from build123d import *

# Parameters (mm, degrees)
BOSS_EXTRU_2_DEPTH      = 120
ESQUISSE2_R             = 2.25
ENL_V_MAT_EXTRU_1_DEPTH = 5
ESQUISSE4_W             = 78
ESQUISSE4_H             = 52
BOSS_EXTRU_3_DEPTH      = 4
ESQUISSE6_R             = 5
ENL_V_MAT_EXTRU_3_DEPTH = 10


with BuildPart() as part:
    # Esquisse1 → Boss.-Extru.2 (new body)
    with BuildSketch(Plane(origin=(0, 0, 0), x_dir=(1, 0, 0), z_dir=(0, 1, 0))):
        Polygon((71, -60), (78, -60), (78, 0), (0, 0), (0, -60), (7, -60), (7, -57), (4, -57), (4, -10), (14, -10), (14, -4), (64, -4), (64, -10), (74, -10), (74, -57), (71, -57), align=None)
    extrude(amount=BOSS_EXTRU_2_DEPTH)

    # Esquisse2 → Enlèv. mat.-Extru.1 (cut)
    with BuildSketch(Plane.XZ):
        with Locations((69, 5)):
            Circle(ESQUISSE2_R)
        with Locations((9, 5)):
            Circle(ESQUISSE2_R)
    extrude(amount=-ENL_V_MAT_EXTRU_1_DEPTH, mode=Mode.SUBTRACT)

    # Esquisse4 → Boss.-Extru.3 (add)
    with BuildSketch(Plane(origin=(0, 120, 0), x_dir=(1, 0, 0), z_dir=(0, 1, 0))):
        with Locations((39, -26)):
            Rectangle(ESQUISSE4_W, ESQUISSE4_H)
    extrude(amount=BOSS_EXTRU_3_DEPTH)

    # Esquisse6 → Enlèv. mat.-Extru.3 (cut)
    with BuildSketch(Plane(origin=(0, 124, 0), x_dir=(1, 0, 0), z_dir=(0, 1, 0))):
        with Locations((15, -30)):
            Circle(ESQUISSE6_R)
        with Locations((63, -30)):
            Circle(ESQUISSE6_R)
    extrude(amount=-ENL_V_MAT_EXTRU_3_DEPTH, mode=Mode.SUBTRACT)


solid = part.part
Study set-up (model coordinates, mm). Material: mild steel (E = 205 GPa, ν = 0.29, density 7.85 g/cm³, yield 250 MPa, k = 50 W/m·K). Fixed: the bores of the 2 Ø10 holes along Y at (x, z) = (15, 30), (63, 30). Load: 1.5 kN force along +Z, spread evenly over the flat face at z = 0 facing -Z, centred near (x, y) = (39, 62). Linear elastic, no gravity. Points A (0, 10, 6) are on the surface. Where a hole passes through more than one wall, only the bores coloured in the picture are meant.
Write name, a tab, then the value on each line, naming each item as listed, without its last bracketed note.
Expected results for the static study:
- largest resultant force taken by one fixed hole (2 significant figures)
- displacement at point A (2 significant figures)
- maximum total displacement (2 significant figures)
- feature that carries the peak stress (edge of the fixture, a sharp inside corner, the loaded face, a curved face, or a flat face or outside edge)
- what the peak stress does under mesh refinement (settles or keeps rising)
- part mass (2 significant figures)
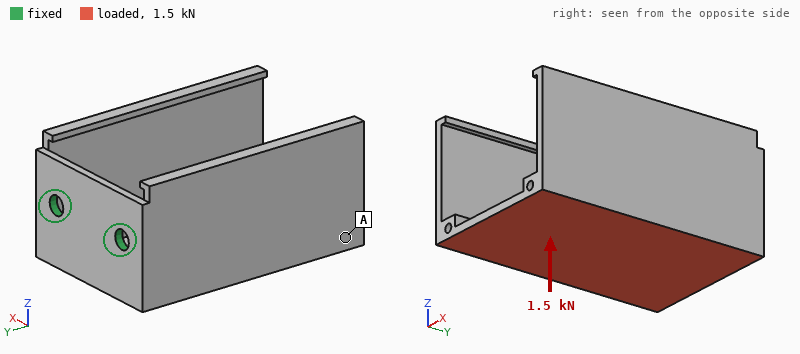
largest resultant force taken by one fixed hole	770 N
displacement at point A	0.37 mm
maximum total displacement	0.45 mm
feature that carries the peak stress	edge of the fixture
what the peak stress does under mesh refinement	keeps rising
part mass	970 g
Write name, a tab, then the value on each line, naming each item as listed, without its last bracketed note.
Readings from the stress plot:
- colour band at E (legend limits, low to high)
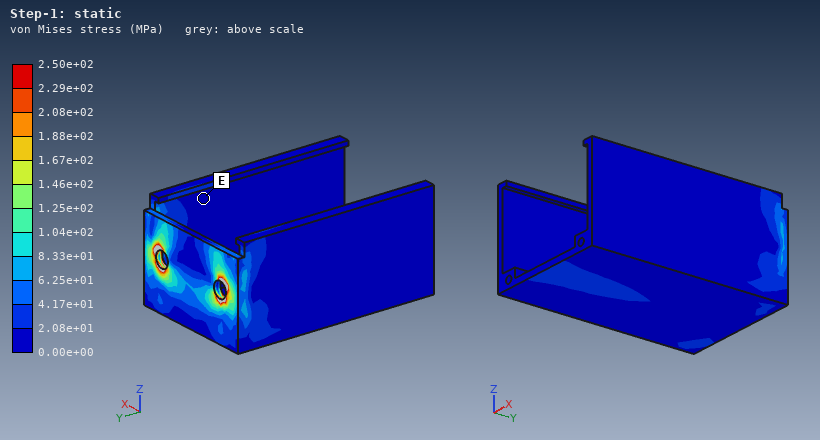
colour band at E	0.00e+00 to 2.08e+01 MPa
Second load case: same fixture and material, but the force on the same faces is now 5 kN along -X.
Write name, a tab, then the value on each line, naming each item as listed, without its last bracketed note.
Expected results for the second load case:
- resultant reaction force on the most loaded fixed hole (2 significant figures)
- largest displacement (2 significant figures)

resultant reaction force on the most loaded fixed hole	5.8 kN
largest displacement	0.72 mm
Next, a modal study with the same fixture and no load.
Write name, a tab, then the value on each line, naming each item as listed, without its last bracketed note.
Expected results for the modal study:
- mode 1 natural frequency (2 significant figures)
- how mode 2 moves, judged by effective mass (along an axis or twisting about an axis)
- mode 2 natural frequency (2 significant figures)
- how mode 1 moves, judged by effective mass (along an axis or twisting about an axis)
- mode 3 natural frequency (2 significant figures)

mode 1 natural frequency	390 Hz
how mode 2 moves, judged by effective mass	along X
mode 2 natural frequency	460 Hz
how mode 1 moves, judged by effective mass	along Z
mode 3 natural frequency	930 Hz
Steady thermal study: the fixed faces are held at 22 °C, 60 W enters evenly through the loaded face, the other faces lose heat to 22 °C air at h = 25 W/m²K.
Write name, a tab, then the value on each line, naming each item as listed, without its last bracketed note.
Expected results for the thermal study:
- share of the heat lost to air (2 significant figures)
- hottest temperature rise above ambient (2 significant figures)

share of the heat lost to air	61 %
hottest temperature rise above ambient	59 K
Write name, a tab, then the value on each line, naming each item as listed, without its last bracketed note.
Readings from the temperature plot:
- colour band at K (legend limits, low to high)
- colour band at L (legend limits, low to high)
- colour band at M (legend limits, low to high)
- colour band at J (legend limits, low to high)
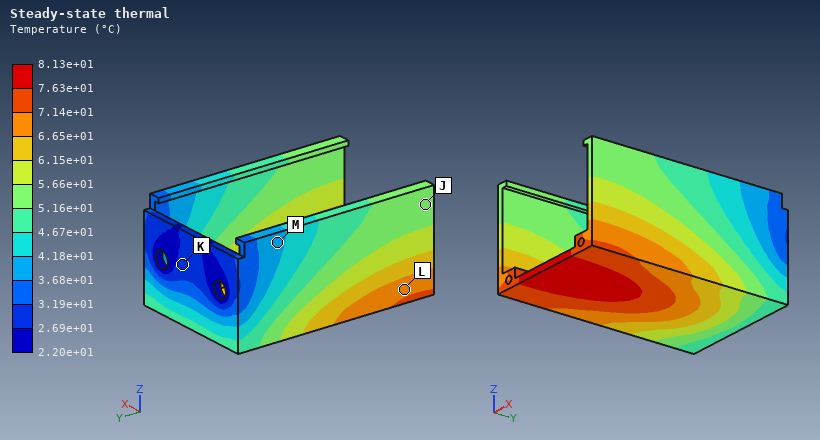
colour band at K	2.69e+01 to 3.19e+01 °C
colour band at L	6.65e+01 to 7.14e+01 °C
colour band at M	3.68e+01 to 4.18e+01 °C
colour band at J	5.16e+01 to 5.66e+01 °C
